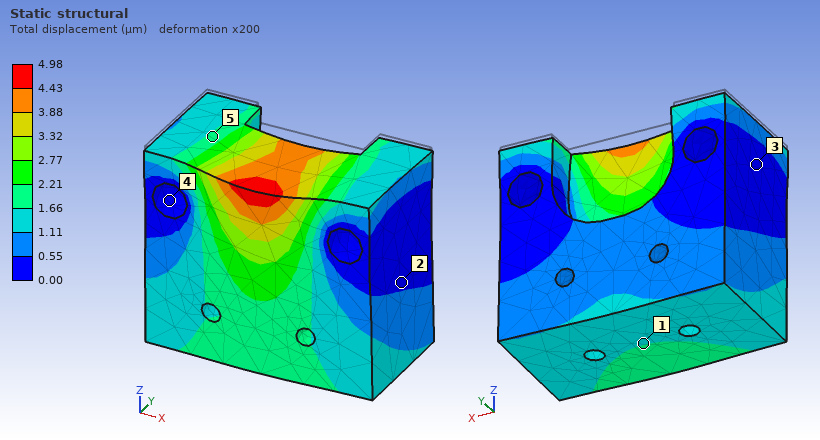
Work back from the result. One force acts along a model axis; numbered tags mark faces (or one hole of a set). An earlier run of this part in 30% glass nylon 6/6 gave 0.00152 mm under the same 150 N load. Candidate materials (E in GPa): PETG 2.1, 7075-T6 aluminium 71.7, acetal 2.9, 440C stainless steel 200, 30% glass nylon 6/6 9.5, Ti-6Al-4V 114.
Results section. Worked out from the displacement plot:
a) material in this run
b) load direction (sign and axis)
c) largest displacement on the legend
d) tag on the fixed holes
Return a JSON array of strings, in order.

["acetal", "-Z", "4.98 µm", "4"]
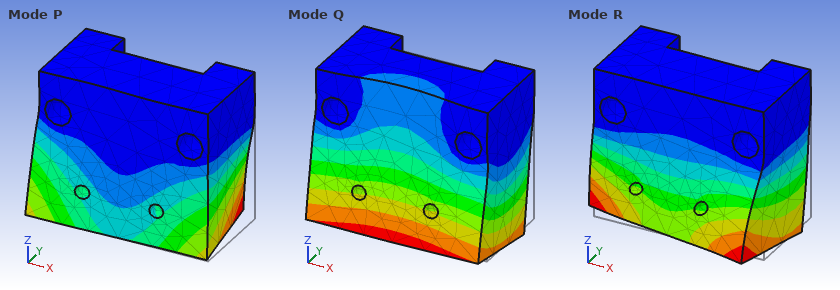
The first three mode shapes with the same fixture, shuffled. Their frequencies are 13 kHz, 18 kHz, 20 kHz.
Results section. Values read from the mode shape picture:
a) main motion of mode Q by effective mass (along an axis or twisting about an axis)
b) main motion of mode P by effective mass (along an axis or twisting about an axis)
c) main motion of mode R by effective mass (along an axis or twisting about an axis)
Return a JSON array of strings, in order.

["along Y", "along X", "along X"]
